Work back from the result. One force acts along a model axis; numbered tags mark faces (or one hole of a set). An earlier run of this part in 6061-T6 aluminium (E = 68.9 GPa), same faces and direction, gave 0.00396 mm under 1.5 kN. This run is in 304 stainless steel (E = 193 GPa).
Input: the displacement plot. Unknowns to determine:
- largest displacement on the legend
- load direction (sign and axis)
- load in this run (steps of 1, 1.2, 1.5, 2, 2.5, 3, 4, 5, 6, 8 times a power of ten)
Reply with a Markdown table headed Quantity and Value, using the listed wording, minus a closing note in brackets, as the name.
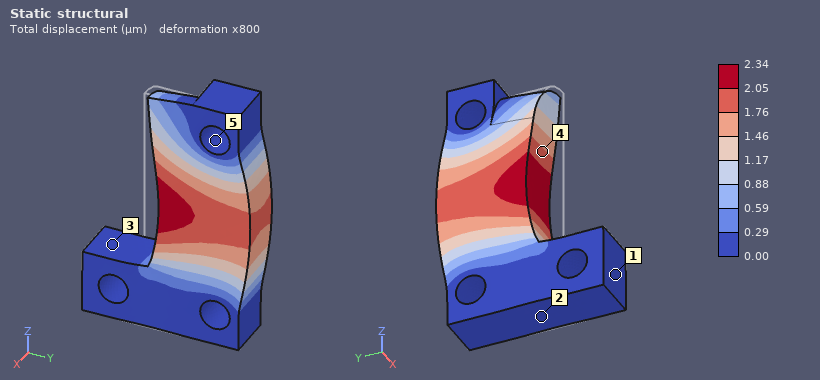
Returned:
| Quantity | Value |
|---|---|
| largest displacement on the legend | 2.34 µm |
| load direction | +Y |
| load in this run | 2.5 kN |
